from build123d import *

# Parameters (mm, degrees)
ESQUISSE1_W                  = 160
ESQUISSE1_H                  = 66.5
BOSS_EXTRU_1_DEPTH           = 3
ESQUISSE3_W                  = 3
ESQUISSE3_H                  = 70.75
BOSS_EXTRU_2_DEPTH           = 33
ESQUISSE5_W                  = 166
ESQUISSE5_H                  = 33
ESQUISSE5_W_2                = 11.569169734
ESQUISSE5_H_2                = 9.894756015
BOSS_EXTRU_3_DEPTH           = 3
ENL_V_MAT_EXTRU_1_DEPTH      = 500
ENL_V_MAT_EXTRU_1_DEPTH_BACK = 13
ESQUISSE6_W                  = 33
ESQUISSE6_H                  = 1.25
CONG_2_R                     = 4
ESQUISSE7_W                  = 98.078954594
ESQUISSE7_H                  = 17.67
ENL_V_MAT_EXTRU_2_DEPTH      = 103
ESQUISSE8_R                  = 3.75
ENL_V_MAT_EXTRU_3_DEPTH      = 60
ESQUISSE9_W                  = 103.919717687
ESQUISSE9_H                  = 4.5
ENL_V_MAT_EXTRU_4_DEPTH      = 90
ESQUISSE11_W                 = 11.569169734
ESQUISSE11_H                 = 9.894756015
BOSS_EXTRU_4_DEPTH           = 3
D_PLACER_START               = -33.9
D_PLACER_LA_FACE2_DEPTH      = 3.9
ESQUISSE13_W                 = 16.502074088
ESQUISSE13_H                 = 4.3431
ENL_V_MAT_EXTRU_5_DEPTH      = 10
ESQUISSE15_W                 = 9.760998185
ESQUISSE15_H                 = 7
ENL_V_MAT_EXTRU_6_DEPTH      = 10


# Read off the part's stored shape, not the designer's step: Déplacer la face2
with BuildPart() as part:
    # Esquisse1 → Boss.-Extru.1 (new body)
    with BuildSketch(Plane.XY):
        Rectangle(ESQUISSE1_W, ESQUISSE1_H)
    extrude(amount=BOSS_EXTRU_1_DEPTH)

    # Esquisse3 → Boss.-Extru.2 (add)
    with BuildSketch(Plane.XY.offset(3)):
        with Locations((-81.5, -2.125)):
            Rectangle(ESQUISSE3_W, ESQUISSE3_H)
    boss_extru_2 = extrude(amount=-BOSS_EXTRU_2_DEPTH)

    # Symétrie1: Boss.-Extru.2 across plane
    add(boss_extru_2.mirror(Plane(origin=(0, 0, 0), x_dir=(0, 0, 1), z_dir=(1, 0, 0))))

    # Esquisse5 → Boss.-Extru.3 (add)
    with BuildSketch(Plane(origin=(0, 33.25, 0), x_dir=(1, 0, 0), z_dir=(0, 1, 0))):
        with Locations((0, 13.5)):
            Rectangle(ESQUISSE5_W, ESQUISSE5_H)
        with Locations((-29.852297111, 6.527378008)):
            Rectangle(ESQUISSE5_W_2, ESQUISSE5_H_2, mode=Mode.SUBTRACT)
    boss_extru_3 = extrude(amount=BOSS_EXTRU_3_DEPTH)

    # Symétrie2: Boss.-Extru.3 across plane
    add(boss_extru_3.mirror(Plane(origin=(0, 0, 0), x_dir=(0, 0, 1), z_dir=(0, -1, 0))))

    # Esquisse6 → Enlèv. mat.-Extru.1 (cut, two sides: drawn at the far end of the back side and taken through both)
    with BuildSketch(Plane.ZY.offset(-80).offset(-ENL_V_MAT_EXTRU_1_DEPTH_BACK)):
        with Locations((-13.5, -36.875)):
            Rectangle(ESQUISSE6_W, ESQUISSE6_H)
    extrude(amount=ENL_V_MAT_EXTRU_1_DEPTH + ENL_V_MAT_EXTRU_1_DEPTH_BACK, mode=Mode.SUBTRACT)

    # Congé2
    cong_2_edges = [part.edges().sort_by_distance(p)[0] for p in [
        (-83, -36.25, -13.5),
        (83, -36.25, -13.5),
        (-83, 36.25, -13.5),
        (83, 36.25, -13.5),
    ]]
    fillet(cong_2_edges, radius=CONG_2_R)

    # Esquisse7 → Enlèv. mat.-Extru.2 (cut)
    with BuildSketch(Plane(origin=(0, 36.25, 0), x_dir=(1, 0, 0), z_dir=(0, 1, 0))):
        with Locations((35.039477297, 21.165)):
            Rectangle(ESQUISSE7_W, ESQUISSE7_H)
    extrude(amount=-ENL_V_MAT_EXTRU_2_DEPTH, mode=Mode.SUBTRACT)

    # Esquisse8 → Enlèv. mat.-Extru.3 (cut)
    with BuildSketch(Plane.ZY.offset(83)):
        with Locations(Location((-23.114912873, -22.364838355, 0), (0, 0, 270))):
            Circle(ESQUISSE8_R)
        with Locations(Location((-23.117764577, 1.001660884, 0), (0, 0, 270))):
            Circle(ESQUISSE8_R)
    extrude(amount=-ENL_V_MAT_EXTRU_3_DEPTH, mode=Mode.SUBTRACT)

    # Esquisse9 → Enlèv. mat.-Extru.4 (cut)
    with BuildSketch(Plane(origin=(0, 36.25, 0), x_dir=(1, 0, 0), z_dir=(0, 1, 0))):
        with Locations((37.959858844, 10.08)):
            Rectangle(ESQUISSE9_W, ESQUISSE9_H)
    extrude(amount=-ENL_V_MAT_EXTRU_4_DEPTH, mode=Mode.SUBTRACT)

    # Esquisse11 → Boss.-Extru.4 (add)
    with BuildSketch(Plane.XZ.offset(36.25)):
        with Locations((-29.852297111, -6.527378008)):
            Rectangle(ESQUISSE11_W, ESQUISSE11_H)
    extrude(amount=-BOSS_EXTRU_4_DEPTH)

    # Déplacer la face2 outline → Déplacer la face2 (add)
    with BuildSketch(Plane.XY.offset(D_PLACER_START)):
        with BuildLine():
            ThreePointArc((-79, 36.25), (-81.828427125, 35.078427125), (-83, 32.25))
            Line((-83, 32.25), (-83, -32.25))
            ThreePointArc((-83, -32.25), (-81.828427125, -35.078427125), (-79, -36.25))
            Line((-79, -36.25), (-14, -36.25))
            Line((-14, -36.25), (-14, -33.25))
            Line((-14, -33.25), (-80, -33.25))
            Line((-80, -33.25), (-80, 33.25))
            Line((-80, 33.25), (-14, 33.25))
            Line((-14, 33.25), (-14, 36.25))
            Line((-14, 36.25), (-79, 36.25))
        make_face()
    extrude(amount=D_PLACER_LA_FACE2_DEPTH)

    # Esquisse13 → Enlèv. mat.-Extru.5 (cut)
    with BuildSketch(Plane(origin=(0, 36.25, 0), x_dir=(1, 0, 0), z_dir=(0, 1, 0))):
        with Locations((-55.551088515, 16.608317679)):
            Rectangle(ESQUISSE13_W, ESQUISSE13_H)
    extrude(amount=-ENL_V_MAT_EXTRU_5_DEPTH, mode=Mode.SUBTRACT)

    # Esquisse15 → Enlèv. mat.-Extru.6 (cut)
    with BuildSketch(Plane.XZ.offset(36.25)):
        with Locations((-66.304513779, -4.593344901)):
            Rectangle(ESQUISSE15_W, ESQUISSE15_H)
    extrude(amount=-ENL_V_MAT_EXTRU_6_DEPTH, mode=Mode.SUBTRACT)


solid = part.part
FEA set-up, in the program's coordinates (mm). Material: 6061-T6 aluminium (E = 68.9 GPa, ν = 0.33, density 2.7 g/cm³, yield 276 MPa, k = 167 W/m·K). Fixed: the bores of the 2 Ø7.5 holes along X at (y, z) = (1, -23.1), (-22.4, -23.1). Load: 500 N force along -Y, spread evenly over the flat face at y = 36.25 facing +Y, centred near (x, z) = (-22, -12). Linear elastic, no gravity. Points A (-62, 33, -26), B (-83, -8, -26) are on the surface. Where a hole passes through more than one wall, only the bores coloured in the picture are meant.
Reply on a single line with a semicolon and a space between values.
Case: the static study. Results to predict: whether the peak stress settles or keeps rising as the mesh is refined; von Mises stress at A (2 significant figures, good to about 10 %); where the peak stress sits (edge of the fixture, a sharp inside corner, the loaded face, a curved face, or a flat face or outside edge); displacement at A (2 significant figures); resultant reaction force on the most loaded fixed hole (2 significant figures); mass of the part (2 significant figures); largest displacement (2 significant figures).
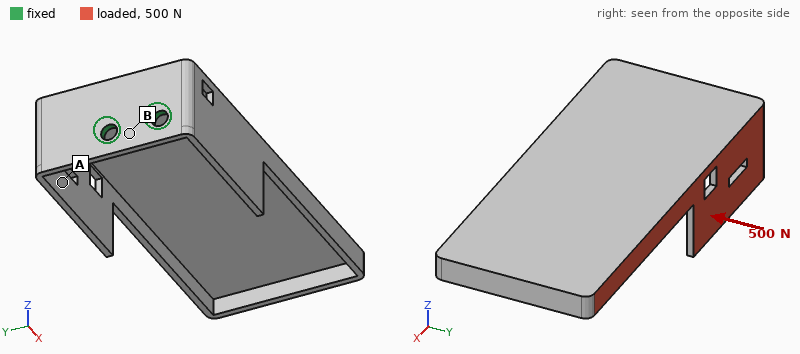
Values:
keeps rising; 39 MPa; edge of the fixture; 0.50 mm; 840 N; 170 g; 2.1 mm
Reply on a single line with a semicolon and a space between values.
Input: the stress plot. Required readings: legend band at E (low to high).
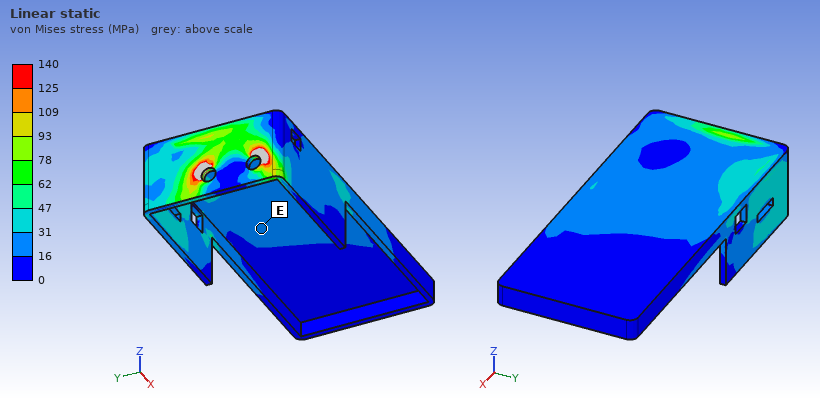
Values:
16 to 31 MPa
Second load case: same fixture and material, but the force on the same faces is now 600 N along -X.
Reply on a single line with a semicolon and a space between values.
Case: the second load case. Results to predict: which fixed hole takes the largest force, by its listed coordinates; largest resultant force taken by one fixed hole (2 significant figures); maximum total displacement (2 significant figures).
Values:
(1, -23.1); 970 N; 1.5 mm
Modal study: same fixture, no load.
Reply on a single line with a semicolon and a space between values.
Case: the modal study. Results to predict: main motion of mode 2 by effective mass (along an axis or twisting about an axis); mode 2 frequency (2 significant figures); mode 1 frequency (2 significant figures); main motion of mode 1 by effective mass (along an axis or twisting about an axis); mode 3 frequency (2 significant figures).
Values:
along Y; 230 Hz; 160 Hz; along Z; 590 Hz
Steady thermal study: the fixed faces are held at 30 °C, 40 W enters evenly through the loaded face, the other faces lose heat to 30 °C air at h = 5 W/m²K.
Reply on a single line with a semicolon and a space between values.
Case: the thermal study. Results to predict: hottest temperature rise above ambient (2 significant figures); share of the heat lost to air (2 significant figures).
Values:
60 K; 18 %
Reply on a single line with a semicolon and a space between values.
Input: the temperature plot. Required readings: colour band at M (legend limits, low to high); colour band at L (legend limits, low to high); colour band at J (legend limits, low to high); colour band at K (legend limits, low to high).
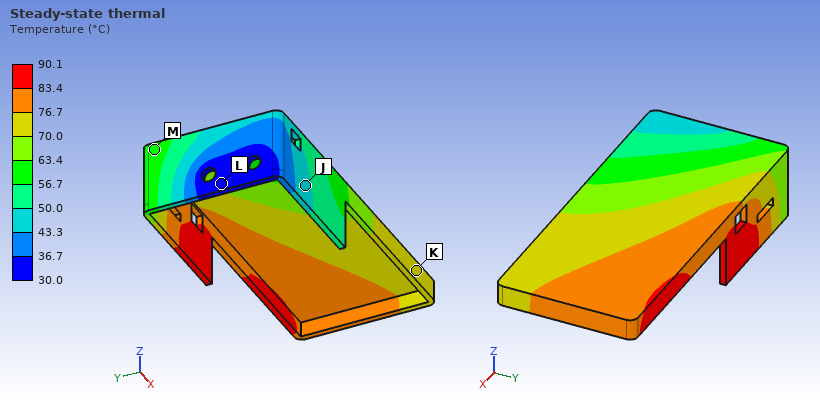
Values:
56.7 to 63.4 °C; 30.0 to 36.7 °C; 43.3 to 50.0 °C; 70.0 to 76.7 °C
